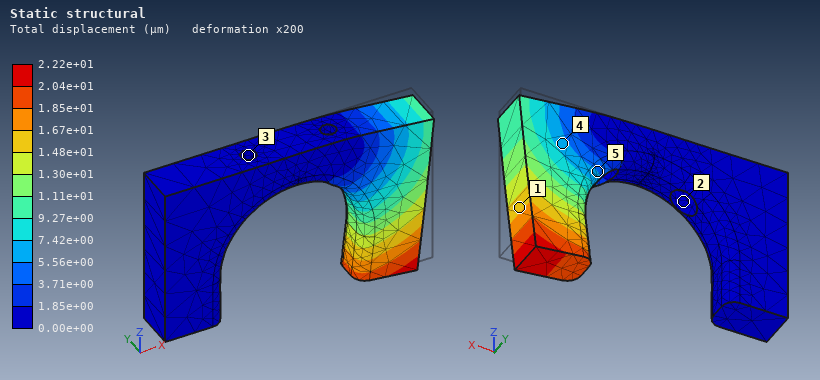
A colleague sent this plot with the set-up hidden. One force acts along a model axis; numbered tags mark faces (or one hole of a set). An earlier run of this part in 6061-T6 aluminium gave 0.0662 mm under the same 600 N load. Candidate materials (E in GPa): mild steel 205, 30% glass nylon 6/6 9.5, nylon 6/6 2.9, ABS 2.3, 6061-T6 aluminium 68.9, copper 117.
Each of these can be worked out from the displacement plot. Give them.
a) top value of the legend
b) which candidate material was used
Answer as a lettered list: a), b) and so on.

a) 2.22e+01 µm
b) mild steel
